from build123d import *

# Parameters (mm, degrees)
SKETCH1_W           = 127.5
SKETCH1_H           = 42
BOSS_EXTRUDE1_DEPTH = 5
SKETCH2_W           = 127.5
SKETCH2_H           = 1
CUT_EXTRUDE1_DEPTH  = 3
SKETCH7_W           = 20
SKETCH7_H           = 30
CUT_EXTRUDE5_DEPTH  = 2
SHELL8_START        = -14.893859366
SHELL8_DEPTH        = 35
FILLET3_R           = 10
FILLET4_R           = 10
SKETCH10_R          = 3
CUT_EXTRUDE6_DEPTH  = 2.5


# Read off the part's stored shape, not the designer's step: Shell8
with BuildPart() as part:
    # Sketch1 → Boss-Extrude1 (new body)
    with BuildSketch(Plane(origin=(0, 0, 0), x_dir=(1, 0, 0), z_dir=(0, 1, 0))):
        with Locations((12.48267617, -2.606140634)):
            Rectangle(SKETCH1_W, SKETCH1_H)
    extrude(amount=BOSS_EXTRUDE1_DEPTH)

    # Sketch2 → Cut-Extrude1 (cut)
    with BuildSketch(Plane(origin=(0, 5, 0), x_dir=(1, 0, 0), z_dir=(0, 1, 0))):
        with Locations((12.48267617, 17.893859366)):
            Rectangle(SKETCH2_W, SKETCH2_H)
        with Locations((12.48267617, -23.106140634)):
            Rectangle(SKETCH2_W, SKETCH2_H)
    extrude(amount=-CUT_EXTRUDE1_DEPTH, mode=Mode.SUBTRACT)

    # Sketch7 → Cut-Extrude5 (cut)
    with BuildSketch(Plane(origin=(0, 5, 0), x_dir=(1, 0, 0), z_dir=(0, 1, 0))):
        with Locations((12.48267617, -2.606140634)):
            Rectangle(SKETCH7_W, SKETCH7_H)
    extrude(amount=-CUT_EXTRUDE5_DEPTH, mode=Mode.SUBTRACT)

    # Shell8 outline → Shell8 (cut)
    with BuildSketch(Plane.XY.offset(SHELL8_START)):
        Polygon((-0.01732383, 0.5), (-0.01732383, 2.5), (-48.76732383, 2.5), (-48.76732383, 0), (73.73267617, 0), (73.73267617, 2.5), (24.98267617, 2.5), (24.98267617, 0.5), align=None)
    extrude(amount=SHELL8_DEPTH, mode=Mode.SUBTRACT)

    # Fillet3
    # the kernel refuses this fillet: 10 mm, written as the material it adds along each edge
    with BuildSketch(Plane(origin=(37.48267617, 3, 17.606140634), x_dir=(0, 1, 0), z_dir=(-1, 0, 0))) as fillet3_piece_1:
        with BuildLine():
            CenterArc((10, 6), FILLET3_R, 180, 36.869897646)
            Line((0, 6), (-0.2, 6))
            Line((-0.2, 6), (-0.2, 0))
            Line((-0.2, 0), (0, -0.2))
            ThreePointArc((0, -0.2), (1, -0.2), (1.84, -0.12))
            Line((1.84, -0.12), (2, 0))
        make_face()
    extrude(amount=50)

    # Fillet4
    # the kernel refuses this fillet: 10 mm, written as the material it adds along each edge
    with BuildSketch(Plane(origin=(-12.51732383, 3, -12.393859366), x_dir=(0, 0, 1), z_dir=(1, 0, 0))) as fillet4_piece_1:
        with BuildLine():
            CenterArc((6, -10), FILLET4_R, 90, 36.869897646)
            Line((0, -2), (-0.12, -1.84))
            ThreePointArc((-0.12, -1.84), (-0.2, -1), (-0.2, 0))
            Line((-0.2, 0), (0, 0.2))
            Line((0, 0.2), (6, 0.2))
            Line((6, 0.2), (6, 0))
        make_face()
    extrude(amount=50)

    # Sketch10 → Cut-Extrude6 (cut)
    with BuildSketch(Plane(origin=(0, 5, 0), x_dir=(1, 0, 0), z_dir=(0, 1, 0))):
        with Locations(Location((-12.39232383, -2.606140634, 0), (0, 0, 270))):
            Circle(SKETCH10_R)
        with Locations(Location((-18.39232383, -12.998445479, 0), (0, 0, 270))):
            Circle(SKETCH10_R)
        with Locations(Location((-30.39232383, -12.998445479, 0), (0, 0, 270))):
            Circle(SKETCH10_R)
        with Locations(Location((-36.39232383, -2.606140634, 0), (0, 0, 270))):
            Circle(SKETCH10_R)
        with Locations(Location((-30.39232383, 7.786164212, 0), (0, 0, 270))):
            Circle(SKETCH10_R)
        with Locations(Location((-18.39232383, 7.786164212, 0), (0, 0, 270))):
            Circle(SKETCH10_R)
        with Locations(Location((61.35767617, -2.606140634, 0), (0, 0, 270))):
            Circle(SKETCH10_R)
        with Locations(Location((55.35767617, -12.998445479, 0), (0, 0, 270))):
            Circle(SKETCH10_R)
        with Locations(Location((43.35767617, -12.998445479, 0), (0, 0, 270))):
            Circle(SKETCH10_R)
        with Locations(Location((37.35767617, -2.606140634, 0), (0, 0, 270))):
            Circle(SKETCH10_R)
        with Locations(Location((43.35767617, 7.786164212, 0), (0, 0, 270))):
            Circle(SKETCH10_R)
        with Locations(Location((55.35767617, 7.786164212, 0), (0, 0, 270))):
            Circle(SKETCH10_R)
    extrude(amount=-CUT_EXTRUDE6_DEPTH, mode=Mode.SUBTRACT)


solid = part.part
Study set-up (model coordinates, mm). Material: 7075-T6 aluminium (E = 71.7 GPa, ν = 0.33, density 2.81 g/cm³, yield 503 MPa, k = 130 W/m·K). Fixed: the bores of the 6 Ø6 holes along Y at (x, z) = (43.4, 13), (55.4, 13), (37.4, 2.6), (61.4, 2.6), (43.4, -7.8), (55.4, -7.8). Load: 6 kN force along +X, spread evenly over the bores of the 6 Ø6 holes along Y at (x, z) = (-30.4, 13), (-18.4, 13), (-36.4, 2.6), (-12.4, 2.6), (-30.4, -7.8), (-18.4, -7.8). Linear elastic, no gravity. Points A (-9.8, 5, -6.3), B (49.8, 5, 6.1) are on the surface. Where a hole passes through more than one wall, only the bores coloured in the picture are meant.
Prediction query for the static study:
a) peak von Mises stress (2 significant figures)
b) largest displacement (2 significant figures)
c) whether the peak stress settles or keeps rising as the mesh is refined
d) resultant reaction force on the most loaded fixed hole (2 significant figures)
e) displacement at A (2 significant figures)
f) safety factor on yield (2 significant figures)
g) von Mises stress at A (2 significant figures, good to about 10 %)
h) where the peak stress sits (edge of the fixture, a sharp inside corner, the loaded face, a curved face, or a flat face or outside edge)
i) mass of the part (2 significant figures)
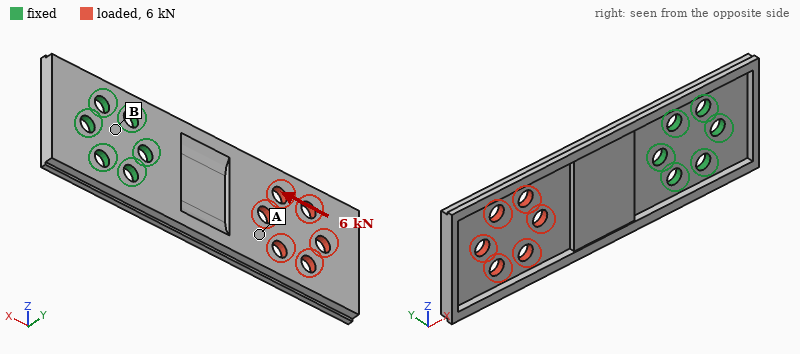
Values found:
200 MPa
1.6 mm
settles
1.9 kN
0.52 mm
2.5
72 MPa
a curved face
43 g
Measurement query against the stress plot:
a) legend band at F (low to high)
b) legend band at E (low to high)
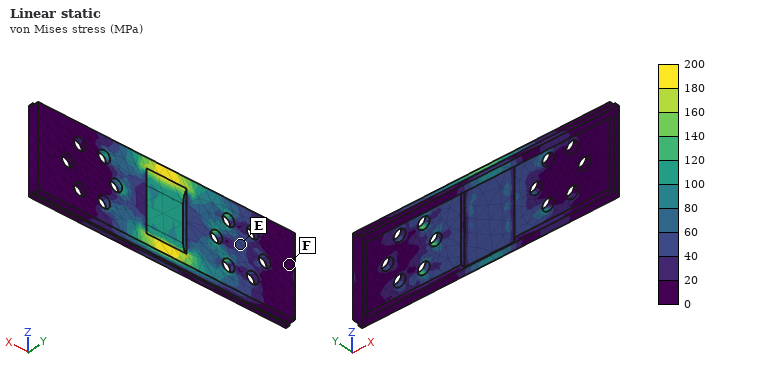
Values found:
0 to 20 MPa
40 to 60 MPa
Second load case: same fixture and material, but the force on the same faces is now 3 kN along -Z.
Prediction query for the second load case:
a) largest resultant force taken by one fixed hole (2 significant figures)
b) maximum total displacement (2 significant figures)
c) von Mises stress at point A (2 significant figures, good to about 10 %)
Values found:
4.5 kN
0.58 mm
83 MPa
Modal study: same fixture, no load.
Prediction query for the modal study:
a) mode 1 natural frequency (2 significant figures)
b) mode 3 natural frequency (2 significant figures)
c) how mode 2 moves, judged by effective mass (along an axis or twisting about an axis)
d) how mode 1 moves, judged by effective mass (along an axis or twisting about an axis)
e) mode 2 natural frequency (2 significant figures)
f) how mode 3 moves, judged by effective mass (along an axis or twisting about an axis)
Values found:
380 Hz
2100 Hz
twisting about X
along Y
1200 Hz
along Y
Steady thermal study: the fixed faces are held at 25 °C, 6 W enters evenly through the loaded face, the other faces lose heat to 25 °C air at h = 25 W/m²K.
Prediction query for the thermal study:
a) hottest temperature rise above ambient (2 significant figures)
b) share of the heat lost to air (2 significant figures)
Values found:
17 K
39 %
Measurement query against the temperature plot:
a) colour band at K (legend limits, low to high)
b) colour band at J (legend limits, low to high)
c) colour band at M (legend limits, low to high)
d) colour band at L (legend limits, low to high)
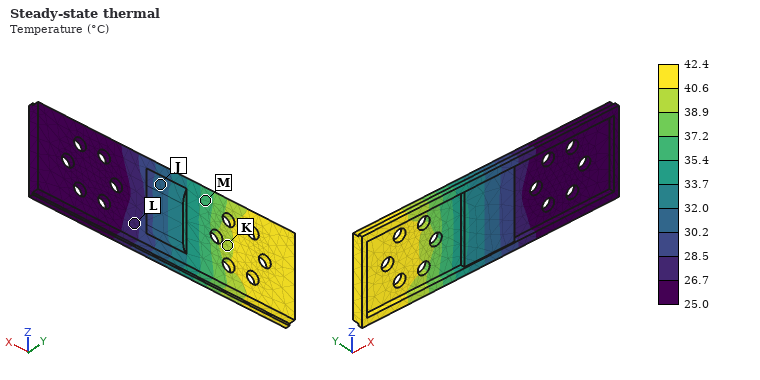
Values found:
38.9 to 40.6 °C
30.2 to 32.0 °C
35.4 to 37.2 °C
26.7 to 28.5 °C
